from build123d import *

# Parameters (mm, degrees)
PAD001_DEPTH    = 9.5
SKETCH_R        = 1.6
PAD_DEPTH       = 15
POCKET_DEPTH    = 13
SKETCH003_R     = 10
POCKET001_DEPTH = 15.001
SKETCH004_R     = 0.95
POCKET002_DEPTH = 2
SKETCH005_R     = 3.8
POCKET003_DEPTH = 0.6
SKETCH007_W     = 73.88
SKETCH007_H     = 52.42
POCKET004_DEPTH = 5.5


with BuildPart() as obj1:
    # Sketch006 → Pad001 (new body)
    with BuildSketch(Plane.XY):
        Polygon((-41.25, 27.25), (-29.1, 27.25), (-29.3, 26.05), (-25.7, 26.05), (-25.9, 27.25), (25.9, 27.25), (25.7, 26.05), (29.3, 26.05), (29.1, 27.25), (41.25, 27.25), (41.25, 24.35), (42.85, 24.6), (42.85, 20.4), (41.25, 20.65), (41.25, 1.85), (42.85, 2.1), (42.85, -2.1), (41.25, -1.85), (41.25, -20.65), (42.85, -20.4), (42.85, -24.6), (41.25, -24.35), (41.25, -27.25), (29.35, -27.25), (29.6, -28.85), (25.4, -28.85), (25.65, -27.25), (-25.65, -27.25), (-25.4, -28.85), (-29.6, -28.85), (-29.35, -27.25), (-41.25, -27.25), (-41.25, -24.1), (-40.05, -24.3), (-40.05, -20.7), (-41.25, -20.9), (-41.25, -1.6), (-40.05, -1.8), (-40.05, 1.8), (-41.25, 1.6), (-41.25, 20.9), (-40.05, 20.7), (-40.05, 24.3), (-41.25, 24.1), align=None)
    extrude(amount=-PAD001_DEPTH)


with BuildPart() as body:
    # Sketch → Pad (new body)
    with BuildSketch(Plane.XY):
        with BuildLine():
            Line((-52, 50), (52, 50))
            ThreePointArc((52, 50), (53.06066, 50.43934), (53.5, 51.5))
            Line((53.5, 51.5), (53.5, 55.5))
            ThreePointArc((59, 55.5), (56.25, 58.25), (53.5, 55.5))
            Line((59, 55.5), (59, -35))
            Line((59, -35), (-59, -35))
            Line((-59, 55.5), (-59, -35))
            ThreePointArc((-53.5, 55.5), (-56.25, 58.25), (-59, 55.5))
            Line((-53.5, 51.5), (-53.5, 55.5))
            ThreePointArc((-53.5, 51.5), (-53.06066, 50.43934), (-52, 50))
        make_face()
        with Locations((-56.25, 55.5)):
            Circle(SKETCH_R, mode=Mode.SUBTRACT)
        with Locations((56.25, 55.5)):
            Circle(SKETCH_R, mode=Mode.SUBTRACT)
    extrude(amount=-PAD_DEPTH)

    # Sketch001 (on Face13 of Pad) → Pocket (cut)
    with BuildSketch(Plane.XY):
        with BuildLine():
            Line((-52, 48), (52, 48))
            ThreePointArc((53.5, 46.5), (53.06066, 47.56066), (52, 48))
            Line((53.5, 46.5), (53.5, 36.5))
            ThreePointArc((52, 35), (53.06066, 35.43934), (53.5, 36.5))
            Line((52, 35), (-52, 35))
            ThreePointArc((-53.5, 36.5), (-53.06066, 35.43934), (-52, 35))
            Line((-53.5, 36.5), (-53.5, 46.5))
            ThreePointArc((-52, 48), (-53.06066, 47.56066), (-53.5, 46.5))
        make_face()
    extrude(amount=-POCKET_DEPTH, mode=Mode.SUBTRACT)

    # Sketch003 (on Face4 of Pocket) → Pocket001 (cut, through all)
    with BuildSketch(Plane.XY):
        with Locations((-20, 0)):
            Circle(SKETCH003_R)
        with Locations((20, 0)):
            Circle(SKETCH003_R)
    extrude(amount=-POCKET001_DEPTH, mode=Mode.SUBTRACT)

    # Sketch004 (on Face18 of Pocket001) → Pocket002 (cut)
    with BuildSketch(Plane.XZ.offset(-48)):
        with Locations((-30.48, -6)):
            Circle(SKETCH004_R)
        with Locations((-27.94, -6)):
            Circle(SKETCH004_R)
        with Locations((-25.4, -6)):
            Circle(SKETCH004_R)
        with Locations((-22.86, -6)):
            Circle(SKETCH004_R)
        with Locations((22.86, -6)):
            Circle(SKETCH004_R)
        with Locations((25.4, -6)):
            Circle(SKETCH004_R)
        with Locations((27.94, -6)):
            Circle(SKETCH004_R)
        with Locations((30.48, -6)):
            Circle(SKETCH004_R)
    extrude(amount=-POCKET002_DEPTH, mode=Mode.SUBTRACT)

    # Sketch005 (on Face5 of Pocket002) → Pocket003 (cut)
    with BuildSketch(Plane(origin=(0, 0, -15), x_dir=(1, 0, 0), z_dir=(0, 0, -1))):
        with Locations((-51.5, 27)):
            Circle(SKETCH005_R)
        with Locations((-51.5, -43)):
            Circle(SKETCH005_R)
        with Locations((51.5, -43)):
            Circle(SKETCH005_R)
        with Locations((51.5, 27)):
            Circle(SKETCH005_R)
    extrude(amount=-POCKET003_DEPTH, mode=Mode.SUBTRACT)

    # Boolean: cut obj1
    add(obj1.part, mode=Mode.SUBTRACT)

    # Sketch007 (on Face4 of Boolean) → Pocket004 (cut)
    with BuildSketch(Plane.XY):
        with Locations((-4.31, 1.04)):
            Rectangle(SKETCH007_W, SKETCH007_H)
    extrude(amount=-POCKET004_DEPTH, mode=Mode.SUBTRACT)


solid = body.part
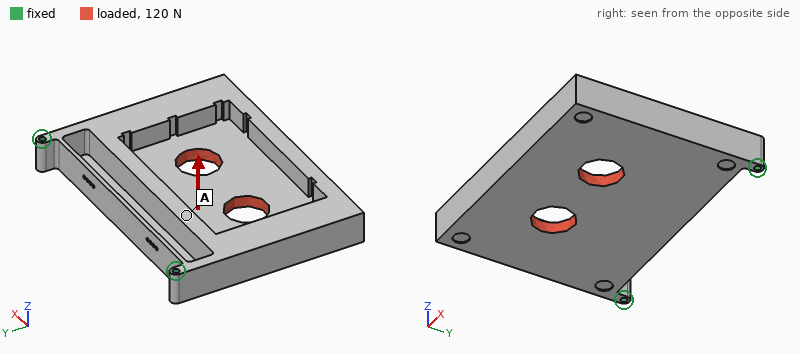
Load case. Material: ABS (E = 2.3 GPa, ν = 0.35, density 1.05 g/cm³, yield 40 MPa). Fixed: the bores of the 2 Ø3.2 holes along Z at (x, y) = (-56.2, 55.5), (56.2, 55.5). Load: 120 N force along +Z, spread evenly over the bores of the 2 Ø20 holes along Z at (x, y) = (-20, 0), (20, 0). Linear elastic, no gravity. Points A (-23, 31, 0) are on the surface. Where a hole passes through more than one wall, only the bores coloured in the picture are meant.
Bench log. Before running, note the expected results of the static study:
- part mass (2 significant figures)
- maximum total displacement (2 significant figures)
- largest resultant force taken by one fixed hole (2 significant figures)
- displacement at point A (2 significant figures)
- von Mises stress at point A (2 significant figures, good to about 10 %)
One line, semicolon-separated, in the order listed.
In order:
91 g; 1.5 mm; 70 N; 0.36 mm; 2.3 MPa
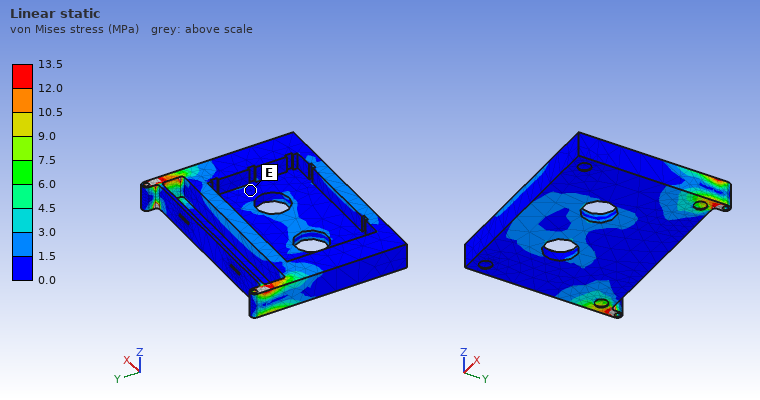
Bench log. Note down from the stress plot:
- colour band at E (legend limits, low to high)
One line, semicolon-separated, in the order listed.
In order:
0.0 to 1.5 MPa
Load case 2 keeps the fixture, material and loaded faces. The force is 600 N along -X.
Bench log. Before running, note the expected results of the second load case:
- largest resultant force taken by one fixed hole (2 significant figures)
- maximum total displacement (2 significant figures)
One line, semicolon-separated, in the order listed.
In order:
400 N; 0.31 mm
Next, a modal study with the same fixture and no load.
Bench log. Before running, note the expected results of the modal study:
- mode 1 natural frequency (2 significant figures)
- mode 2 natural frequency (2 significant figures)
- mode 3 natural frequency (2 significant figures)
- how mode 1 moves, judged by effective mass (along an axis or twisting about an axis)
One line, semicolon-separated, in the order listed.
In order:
190 Hz; 420 Hz; 910 Hz; along Z
